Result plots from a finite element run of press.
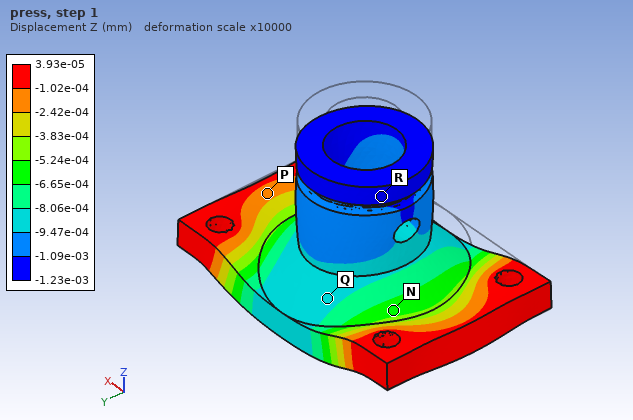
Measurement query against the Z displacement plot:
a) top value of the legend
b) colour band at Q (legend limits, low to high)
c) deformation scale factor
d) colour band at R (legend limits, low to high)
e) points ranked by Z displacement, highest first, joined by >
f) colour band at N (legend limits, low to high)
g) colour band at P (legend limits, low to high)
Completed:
3.93e-05 mm
-9.47e-04 to -8.06e-04 mm
10000
-1.23e-03 to -1.09e-03 mm
P > N > Q > R
-6.65e-04 to -5.24e-04 mm
-2.42e-04 to -1.02e-04 mm
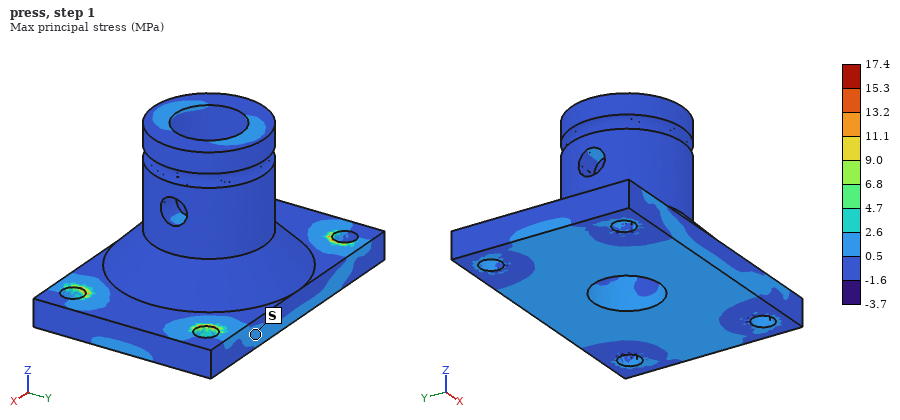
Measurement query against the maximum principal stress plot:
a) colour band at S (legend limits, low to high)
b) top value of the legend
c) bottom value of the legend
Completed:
0.5 to 2.6 MPa
17.4 MPa
-3.7 MPa
